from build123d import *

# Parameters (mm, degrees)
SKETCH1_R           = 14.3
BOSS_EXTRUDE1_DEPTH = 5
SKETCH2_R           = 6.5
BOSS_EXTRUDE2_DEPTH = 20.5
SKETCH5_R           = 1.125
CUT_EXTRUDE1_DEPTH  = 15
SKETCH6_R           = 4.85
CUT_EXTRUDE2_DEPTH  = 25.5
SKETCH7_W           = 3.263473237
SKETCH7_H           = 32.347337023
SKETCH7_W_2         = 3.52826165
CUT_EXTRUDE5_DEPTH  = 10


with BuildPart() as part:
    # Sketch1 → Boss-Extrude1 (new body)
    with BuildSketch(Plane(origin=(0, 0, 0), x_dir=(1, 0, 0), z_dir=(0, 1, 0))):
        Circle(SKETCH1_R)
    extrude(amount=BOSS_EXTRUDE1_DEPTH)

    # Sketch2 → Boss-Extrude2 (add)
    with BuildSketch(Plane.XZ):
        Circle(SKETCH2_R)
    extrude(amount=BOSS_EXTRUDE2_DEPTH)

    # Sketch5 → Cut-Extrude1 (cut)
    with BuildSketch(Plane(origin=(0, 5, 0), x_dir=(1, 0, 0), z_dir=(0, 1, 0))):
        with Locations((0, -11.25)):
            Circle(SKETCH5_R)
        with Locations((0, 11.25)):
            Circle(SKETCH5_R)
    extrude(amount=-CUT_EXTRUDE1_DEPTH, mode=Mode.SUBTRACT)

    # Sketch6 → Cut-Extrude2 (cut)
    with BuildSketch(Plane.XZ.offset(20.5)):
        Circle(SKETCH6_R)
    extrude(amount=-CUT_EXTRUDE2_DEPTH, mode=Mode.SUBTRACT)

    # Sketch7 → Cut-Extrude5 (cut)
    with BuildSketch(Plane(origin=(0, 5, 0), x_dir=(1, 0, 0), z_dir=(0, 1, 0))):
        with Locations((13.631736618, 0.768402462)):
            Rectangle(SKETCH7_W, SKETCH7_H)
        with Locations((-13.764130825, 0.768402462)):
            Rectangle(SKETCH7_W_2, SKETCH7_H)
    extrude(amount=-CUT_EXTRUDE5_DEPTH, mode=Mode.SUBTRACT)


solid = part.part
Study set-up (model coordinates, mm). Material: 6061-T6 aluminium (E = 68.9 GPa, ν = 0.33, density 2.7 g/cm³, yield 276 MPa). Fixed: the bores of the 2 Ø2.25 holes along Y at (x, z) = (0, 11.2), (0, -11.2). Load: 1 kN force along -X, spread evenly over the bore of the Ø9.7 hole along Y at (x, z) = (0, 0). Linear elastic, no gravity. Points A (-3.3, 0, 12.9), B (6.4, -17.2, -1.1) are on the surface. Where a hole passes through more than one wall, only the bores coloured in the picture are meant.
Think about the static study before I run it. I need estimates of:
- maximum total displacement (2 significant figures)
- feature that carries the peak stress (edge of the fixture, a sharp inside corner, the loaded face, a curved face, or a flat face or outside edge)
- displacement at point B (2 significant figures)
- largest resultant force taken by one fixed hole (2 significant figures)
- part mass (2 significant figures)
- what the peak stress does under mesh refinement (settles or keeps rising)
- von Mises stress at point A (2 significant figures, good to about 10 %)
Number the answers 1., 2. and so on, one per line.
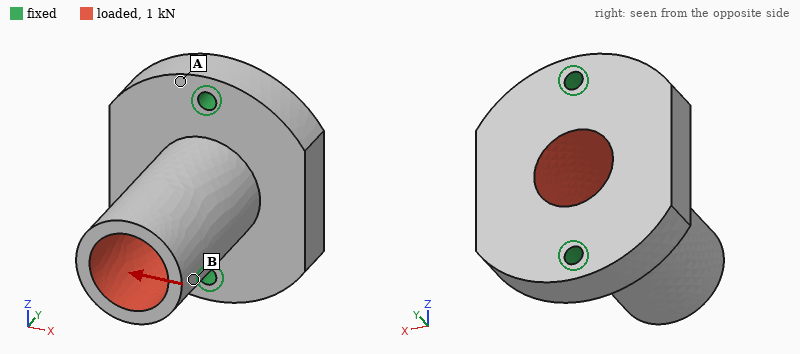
1. 0.10 mm
2. edge of the fixture
3. 0.088 mm
4. 500 N
5. 10 g
6. keeps rising
7. 50 MPa
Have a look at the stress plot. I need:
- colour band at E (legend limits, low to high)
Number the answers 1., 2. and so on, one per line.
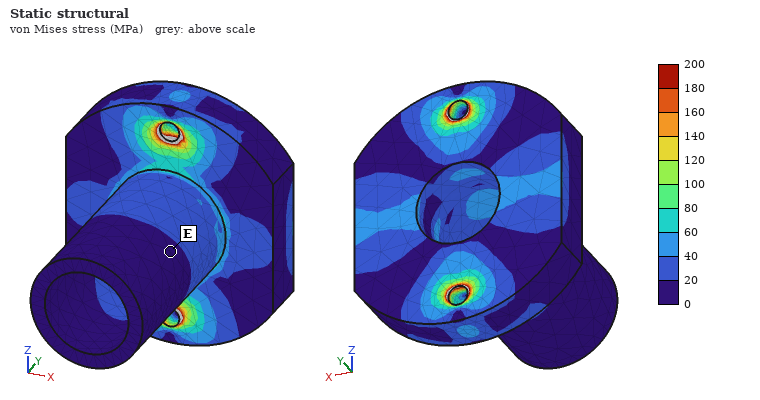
1. 0 to 20 MPa
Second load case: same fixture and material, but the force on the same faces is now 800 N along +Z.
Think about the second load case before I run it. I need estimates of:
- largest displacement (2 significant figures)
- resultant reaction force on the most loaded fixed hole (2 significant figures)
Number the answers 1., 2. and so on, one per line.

1. 33 µm
2. 600 N
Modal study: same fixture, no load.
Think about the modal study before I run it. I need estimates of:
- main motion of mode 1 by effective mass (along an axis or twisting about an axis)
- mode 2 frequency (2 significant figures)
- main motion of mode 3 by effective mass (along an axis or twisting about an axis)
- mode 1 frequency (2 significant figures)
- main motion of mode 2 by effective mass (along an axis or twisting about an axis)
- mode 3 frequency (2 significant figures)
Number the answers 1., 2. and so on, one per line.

1. along X
2. 14 kHz
3. along Y
4. 8600 Hz
5. along Z
6. 21 kHz
